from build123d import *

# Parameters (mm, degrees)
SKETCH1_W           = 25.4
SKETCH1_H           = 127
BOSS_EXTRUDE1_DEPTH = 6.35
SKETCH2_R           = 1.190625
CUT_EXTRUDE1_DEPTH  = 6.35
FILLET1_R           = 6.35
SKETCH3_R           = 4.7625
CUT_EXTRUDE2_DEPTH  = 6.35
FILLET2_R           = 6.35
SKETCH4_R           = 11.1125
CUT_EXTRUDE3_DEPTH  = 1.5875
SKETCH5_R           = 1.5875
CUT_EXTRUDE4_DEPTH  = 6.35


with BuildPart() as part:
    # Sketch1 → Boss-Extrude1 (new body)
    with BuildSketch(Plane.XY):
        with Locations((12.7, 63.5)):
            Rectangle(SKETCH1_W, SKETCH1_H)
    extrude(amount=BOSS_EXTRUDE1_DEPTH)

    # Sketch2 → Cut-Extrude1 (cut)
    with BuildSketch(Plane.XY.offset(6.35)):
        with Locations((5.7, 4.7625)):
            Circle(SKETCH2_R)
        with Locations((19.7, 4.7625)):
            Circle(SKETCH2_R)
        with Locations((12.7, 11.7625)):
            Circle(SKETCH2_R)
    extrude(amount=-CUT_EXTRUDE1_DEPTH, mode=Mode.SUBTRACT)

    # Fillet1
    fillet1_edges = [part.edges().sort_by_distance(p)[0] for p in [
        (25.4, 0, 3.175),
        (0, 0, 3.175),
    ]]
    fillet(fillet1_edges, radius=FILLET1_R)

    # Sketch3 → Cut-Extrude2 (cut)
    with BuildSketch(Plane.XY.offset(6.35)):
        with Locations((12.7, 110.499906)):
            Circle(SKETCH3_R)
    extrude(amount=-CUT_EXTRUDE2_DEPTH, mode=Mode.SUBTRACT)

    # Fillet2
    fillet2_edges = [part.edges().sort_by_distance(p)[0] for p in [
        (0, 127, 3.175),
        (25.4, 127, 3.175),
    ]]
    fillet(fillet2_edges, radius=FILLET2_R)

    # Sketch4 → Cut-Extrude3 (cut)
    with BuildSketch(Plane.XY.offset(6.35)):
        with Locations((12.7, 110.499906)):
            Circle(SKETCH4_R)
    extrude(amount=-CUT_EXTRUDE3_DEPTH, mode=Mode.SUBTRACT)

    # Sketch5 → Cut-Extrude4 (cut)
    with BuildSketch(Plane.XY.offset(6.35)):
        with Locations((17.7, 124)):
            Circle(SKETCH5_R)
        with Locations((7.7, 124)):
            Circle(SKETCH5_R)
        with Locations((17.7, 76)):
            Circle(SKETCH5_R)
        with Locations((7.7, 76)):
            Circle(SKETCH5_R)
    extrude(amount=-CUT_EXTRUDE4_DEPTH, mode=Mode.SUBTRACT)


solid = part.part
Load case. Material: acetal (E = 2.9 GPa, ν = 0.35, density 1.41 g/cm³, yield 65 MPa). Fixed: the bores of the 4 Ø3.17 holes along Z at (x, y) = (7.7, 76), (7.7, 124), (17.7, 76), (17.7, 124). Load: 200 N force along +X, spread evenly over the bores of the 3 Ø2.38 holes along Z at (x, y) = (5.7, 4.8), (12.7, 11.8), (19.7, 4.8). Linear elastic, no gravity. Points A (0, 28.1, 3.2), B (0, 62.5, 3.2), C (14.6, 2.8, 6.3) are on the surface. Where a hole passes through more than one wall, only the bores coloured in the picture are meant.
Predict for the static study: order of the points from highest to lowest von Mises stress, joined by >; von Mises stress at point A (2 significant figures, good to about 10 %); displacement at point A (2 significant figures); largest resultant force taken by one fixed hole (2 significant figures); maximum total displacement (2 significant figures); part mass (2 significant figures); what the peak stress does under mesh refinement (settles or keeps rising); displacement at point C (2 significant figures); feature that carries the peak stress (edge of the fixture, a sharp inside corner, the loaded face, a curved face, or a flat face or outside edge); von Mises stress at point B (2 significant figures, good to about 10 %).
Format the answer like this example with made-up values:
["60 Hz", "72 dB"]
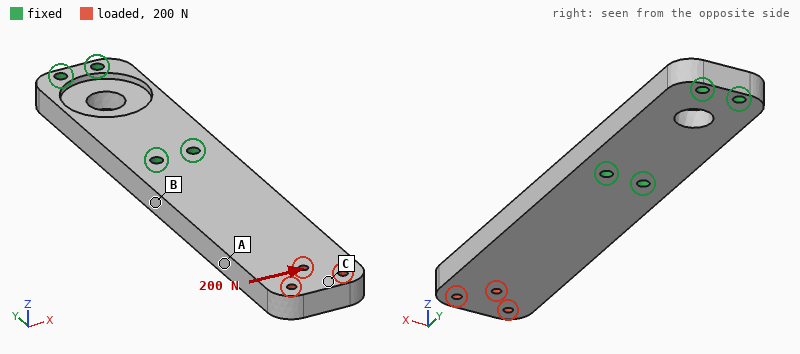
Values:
["B > A > C", "6.1 MPa", "0.73 mm", "880 N", "1.3 mm", "27 g", "keeps rising", "1.3 mm", "edge of the fixture", "16 MPa"]
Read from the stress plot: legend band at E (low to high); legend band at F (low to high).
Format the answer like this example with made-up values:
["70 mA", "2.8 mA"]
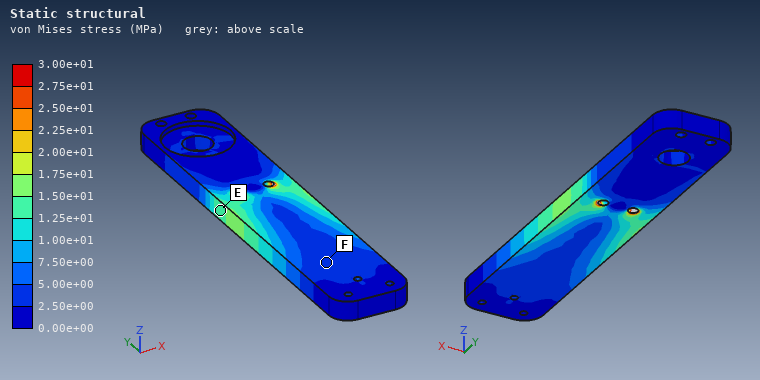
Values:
["1.25e+01 to 1.50e+01 MPa", "2.50e+00 to 5.00e+00 MPa"]
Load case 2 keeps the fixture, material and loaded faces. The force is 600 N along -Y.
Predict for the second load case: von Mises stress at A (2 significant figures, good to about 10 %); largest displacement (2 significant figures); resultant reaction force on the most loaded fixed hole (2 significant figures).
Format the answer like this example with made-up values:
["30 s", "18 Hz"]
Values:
["3.6 MPa", "97 µm", "290 N"]
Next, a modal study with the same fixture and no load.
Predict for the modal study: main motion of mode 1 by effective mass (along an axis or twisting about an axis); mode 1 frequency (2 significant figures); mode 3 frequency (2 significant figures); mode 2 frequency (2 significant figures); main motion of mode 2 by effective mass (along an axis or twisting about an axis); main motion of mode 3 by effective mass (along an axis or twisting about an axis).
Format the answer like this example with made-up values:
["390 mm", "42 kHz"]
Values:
["along Z", "260 Hz", "1400 Hz", "860 Hz", "along X", "twisting about Y"]
